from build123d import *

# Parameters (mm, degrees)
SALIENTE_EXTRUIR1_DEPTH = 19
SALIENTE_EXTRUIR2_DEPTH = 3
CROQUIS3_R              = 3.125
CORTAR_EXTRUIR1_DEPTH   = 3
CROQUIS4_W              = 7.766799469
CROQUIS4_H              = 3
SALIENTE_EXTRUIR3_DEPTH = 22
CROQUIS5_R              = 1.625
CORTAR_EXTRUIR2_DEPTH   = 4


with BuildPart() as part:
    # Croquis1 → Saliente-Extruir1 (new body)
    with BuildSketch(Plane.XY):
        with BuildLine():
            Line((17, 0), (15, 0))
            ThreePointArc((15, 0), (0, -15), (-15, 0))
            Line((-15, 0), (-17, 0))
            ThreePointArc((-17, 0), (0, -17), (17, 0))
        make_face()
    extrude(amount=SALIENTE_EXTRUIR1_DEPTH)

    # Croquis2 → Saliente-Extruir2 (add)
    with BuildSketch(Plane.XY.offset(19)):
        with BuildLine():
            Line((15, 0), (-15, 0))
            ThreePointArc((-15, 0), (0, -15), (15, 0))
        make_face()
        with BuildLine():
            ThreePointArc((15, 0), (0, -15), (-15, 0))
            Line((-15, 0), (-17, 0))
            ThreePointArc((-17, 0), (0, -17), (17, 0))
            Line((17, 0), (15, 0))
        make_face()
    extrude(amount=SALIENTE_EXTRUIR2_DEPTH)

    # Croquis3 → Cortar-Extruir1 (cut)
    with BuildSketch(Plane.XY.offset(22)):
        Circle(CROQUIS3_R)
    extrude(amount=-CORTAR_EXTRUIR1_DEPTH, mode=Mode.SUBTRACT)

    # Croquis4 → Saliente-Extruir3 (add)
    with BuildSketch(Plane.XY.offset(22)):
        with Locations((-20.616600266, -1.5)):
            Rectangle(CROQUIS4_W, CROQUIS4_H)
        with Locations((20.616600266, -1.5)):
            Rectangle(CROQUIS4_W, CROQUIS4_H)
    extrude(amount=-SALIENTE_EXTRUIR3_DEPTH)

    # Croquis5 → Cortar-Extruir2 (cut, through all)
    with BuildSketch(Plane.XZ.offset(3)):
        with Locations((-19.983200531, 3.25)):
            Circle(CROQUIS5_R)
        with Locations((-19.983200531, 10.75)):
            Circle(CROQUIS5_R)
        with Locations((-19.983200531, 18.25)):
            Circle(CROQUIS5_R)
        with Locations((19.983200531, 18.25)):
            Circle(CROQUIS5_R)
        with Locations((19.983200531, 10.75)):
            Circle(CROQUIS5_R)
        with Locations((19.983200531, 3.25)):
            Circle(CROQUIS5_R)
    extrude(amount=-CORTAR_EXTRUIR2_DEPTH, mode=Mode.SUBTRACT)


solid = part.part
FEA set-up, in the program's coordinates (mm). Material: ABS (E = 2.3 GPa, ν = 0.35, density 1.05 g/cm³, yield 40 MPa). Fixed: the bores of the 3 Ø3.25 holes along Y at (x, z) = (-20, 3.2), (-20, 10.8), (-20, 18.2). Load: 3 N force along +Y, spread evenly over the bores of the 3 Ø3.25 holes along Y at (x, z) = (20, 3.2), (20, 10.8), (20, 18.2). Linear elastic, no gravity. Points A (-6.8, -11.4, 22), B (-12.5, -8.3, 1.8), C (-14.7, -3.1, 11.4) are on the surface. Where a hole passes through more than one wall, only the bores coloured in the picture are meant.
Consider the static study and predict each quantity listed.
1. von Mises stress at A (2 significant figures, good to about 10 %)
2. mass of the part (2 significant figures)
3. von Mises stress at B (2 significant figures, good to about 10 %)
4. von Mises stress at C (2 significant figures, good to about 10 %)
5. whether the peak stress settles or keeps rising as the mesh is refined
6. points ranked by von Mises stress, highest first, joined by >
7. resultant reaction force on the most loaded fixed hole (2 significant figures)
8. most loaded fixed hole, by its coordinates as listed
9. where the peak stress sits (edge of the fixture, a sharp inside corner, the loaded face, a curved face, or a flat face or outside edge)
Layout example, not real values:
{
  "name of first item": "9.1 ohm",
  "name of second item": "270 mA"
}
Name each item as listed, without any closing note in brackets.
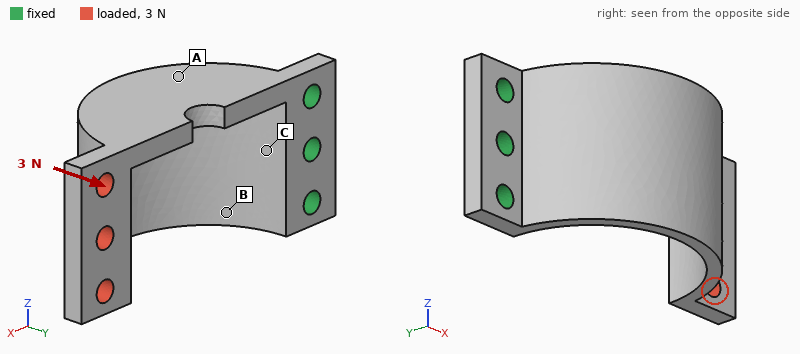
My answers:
{
  "von Mises stress at A": "0.78 MPa",
  "mass of the part": "4.3 g",
  "von Mises stress at B": "2.5 MPa",
  "von Mises stress at C": "3.6 MPa",
  "whether the peak stress settles or keeps rising as the mesh is refined": "keeps rising",
  "points ranked by von Mises stress, highest first, joined by >": "C > B > A",
  "resultant reaction force on the most loaded fixed hole": "3.1 N",
  "most loaded fixed hole, by its coordinates as listed": "(-20, 10.8)",
  "where the peak stress sits": "edge of the fixture"
}
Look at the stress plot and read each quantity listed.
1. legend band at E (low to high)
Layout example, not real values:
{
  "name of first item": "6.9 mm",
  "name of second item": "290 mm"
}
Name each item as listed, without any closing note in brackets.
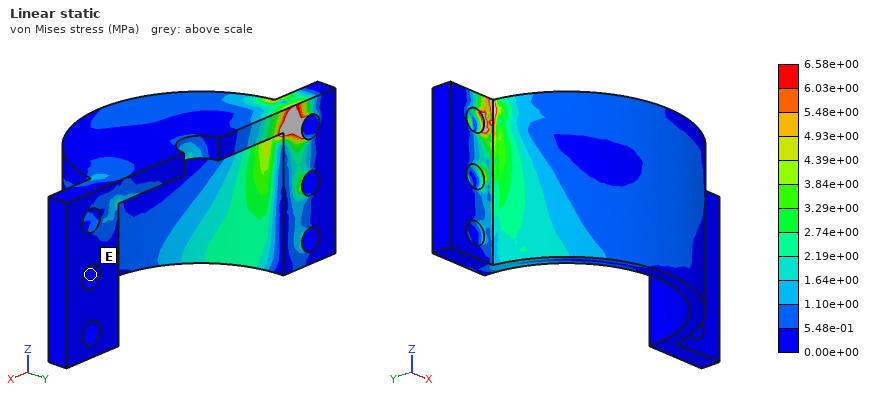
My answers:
{
  "legend band at E": "0.00e+00 to 5.48e-01 MPa"
}
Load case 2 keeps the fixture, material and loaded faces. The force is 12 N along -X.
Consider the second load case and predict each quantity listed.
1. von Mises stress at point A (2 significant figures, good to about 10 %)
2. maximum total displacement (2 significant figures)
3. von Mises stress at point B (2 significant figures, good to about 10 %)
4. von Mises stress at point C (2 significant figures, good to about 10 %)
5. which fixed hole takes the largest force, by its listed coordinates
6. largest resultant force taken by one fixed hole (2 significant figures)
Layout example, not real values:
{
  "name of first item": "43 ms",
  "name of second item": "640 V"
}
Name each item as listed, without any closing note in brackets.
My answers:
{
  "von Mises stress at point A": "1.6 MPa",
  "maximum total displacement": "0.65 mm",
  "von Mises stress at point B": "2.4 MPa",
  "von Mises stress at point C": "1.1 MPa",
  "which fixed hole takes the largest force, by its listed coordinates": "(-20, 18.2)",
  "largest resultant force taken by one fixed hole": "5.2 N"
}
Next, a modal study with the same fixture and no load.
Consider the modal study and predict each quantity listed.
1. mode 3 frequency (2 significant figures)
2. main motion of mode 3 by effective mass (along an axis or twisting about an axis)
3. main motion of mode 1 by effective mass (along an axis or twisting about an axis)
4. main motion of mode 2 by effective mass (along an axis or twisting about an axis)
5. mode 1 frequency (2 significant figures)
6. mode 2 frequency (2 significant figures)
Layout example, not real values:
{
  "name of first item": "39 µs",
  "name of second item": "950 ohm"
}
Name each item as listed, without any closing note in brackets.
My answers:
{
  "mode 3 frequency": "1300 Hz",
  "main motion of mode 3 by effective mass": "along X",
  "main motion of mode 1 by effective mass": "along Y",
  "main motion of mode 2 by effective mass": "along Z",
  "mode 1 frequency": "330 Hz",
  "mode 2 frequency": "450 Hz"
}
